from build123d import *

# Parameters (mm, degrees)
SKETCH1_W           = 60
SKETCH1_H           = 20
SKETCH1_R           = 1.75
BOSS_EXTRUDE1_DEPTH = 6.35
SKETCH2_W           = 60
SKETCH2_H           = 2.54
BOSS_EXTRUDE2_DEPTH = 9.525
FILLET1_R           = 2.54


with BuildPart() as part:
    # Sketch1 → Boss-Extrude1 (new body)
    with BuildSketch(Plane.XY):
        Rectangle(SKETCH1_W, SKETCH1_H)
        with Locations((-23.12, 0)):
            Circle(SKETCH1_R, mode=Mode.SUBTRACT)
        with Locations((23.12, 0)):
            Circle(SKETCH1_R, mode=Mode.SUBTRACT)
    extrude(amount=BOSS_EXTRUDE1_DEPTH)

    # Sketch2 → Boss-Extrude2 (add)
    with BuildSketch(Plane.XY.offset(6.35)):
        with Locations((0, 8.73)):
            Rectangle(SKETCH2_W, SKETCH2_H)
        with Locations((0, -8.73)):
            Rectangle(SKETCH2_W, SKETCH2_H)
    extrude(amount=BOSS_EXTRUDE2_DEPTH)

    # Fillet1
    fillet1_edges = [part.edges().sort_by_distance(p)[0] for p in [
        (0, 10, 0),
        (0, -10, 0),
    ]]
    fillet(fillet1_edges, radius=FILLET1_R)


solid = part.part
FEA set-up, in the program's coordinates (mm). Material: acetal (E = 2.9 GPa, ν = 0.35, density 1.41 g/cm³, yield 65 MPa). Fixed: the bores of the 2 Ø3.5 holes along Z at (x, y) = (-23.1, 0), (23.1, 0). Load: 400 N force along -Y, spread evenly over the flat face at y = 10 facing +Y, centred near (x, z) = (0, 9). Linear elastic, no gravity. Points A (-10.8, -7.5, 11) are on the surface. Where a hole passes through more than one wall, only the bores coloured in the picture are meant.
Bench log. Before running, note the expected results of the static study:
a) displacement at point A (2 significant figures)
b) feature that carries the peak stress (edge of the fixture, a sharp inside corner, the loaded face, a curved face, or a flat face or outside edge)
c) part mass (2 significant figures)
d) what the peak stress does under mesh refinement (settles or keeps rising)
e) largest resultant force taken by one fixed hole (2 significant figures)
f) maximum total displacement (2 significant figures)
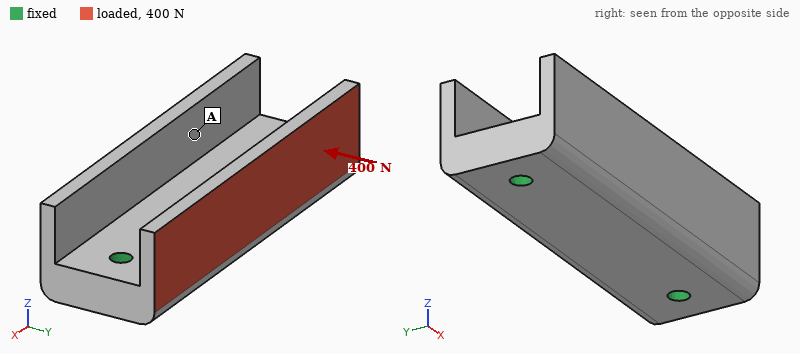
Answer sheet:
0.075 mm
edge of the fixture
14 g
keeps rising
200 N
0.38 mm
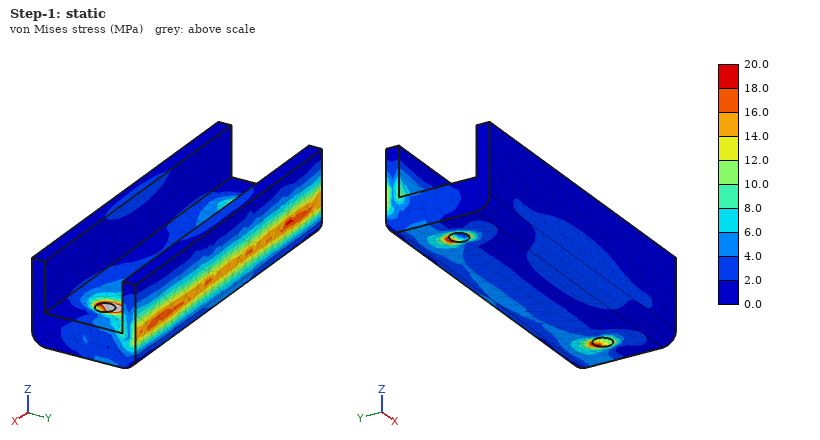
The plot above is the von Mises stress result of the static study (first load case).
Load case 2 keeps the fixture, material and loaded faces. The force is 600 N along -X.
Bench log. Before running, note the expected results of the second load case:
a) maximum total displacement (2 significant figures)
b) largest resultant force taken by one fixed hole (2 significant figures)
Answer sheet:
78 µm
330 N
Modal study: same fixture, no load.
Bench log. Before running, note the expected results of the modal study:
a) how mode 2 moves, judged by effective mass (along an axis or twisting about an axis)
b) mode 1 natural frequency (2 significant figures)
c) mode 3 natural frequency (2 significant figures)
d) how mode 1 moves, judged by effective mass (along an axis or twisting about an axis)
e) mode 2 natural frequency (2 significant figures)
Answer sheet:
along Z
3000 Hz
4500 Hz
along Y
4100 Hz
